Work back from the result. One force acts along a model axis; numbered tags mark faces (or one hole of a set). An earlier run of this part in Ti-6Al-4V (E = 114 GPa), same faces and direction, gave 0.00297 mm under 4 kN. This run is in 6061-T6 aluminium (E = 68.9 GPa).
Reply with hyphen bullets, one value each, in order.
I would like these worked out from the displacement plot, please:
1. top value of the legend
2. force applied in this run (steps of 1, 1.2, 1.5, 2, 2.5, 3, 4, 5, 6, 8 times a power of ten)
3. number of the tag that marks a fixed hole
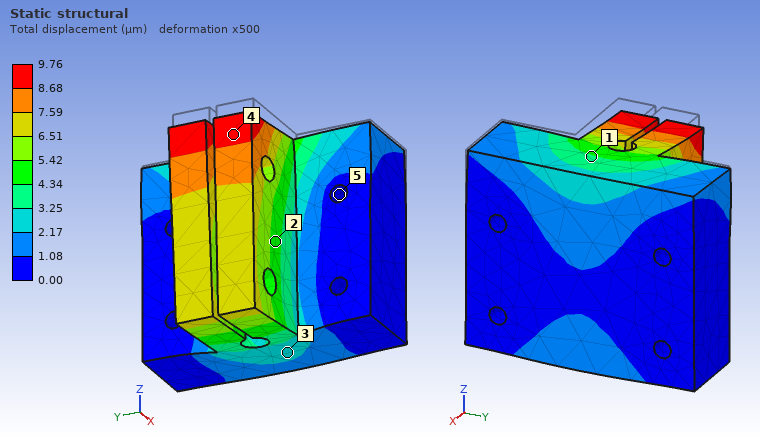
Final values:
- 9.76 µm
- 8 kN
- 5
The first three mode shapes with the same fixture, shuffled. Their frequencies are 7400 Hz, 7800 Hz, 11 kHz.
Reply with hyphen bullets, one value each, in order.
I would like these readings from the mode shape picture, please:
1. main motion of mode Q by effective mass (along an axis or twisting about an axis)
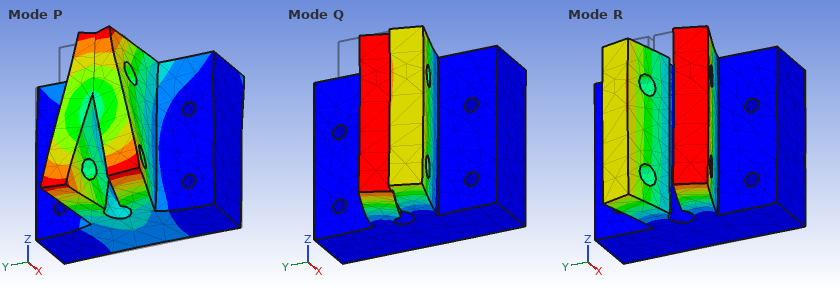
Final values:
- along Y
